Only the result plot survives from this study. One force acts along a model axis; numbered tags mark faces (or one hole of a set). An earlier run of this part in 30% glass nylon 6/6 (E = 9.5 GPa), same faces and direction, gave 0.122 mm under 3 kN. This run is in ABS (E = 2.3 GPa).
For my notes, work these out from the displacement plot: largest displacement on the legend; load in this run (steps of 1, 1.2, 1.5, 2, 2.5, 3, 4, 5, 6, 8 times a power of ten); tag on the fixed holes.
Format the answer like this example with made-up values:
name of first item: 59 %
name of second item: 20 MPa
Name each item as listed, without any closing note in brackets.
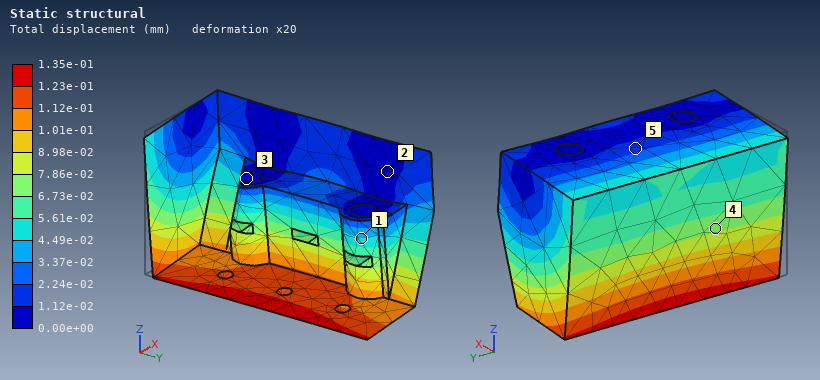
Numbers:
largest displacement on the legend: 1.35e-01 mm
load in this run: 800 N
tag on the fixed holes: 3
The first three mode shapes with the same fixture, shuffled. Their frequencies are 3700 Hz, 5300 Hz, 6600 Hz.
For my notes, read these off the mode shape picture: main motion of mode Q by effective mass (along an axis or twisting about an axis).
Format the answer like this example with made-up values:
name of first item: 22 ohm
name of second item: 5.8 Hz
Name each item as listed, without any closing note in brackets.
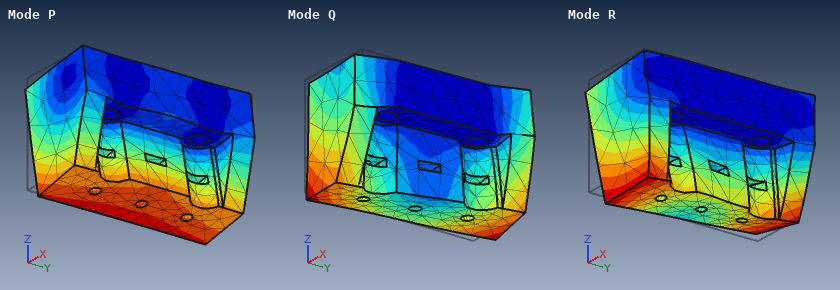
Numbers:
main motion of mode Q by effective mass: along Y
